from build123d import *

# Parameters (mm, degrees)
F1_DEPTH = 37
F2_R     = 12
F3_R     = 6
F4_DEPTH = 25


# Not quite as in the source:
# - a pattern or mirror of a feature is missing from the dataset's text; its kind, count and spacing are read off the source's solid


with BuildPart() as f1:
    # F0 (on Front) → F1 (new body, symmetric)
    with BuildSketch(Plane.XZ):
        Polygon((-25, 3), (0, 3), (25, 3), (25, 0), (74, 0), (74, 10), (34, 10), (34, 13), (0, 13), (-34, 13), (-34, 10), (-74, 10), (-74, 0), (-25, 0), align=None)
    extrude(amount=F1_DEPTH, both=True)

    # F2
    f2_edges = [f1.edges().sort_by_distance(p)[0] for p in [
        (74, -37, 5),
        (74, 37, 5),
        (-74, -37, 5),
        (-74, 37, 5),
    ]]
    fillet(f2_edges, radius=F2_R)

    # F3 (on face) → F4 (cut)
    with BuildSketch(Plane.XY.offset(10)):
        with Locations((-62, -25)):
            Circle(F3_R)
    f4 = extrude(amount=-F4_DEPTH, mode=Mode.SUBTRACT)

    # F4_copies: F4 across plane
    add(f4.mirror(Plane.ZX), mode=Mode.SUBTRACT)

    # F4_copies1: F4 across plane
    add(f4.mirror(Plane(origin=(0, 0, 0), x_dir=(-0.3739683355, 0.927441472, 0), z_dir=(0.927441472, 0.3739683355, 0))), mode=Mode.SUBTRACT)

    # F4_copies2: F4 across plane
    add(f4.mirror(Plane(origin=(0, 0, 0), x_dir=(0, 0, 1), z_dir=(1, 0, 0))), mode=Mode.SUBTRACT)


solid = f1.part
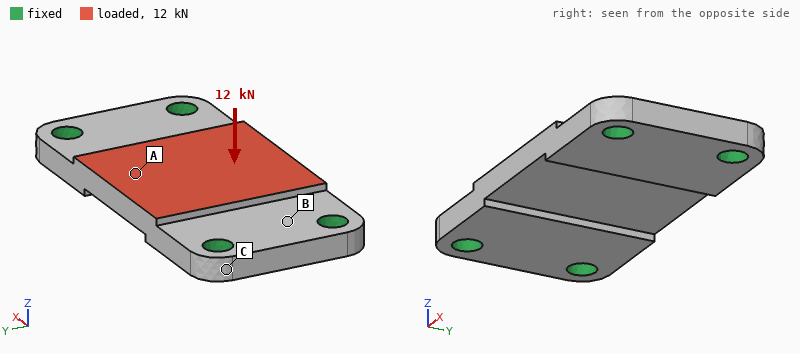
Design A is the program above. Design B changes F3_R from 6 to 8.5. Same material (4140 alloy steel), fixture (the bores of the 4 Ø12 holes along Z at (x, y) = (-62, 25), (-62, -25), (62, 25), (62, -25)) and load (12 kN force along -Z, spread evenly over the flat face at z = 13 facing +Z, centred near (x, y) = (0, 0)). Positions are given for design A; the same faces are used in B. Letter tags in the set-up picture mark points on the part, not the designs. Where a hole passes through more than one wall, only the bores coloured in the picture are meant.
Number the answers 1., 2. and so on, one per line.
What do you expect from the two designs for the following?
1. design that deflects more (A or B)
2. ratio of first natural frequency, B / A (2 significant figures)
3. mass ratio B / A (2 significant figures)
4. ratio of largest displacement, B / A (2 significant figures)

1. A
2. 1.1
3. 0.96
4. 0.83
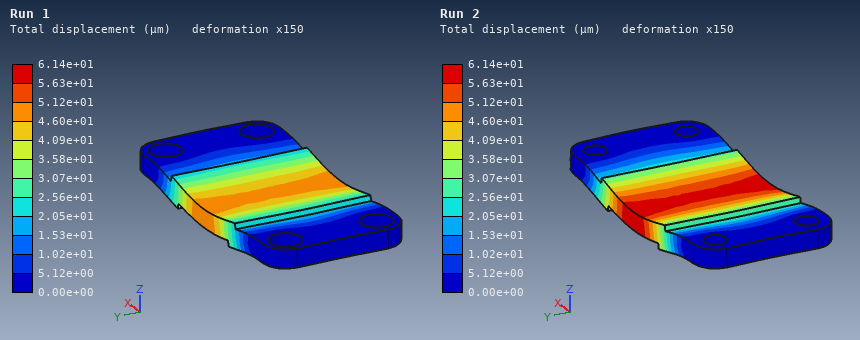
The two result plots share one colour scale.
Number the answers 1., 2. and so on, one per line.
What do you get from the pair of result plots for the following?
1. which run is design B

1. Run 1
